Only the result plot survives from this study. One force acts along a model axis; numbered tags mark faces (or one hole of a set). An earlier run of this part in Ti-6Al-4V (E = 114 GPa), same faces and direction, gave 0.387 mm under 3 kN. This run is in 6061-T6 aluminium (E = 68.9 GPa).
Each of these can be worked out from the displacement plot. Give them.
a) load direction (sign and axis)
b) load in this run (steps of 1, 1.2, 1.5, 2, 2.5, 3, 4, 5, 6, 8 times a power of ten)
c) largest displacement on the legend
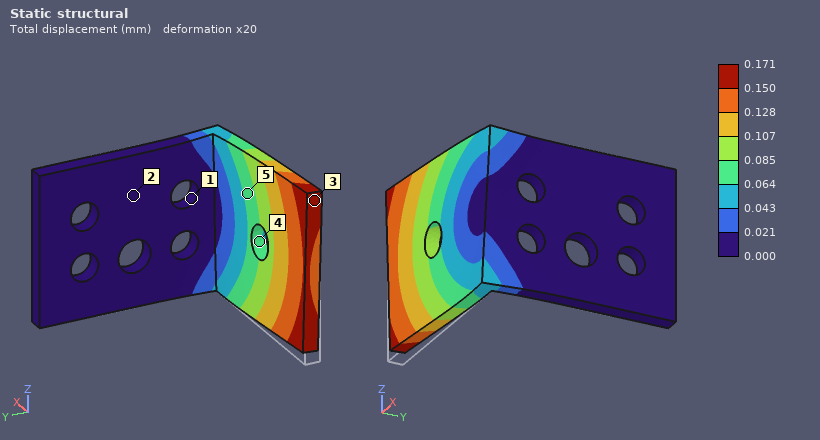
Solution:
+Z
800 N
0.171 mm
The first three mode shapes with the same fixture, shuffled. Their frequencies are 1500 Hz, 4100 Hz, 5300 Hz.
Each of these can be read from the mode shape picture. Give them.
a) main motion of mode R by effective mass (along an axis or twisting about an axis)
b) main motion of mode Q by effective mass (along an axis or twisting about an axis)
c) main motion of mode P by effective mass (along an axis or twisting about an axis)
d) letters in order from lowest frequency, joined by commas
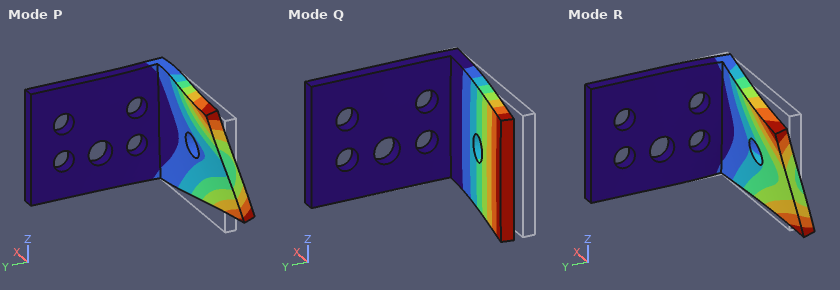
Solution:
along Z
along Y
along Z
Q, R, P
